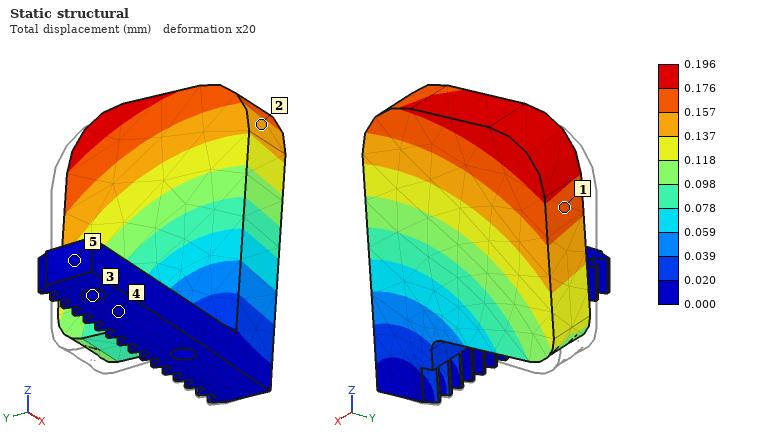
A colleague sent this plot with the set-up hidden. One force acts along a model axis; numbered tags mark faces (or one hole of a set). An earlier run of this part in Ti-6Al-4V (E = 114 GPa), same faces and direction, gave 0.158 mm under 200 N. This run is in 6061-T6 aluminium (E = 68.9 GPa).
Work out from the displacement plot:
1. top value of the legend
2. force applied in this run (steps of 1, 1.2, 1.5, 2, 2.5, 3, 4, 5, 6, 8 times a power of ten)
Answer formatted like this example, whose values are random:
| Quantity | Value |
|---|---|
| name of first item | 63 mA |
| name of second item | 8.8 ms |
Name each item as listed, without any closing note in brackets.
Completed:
| Quantity | Value |
|---|---|
| top value of the legend | 0.196 mm |
| force applied in this run | 150 N |
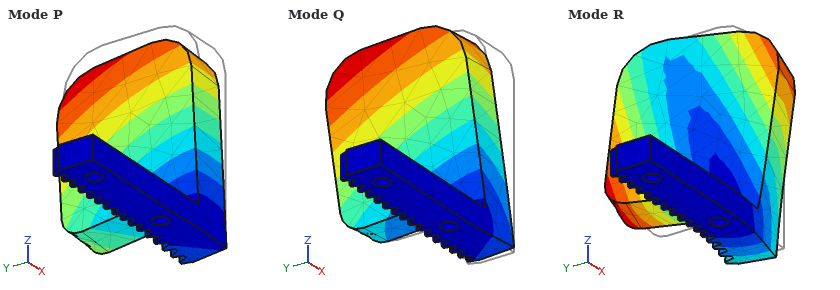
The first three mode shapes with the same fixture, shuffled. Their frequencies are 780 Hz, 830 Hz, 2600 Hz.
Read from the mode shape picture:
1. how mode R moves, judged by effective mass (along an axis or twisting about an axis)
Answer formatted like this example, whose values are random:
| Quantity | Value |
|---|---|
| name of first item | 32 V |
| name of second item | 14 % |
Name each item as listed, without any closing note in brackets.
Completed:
| Quantity | Value |
|---|---|
| how mode R moves, judged by effective mass | twisting about Z |
